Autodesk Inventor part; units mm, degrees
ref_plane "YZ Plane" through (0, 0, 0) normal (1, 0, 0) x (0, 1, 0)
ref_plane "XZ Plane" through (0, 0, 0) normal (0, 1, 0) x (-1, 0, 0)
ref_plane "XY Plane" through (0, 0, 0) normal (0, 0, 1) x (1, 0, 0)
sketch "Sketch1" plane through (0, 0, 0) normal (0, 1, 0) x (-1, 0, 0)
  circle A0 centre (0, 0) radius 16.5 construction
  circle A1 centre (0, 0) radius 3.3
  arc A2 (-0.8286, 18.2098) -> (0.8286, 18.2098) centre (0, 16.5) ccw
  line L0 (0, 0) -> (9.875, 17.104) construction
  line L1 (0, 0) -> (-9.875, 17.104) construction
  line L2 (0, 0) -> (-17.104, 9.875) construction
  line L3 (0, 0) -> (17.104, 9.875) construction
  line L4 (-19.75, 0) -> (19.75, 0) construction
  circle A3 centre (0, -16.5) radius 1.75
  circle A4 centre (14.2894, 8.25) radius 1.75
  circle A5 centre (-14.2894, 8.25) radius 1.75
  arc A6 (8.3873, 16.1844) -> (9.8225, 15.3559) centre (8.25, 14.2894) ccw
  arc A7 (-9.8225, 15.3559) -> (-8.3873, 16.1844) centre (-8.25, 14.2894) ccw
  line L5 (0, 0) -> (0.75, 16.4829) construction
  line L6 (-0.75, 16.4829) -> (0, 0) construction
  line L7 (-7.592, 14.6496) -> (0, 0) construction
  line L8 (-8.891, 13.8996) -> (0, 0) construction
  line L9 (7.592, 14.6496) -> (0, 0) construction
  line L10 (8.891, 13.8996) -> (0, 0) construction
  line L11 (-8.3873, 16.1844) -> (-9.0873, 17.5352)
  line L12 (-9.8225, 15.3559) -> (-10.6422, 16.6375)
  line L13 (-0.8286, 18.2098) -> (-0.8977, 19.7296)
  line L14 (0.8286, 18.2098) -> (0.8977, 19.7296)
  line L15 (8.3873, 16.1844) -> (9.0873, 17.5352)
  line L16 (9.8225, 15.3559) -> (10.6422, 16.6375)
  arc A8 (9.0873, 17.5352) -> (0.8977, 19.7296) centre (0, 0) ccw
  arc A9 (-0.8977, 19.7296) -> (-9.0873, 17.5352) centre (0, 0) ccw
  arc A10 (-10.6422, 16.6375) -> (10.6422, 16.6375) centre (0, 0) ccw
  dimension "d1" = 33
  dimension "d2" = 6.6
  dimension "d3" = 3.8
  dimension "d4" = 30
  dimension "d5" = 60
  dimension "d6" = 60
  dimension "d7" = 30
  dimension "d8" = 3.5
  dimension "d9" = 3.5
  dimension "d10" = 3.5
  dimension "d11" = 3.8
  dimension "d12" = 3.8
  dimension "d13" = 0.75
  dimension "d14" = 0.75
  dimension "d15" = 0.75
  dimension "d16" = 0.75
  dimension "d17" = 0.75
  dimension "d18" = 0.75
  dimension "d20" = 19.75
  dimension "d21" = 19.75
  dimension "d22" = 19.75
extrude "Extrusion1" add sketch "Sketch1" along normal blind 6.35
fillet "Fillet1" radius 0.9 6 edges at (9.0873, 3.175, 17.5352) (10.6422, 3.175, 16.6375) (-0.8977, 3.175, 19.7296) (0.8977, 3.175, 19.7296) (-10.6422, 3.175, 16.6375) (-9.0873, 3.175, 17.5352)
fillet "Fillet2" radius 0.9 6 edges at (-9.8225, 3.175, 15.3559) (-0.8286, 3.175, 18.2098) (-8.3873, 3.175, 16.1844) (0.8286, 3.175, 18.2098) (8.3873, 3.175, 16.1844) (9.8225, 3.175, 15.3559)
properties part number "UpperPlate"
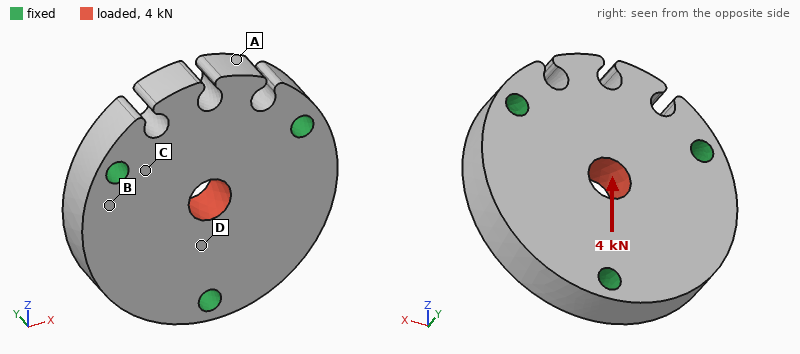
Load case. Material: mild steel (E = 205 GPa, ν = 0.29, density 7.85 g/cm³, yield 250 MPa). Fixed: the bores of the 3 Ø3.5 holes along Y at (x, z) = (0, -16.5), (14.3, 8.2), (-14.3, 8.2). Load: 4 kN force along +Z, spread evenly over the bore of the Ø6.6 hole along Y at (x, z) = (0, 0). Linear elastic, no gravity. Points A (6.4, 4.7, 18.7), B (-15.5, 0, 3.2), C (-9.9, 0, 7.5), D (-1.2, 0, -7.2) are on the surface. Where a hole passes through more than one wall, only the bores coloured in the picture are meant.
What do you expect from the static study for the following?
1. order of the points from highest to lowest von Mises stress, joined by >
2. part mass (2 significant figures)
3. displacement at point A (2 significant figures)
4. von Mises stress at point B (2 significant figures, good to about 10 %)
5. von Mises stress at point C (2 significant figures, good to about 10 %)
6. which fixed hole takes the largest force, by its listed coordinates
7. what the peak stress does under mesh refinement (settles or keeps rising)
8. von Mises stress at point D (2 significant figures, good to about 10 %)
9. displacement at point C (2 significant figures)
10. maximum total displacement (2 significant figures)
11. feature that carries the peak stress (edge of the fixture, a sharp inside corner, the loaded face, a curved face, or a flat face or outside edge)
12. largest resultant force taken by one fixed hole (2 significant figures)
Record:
D > C > B > A
56 g
1.7 µm
13 MPa
21 MPa
(0, -16.5)
keeps rising
32 MPa
0.80 µm
2.8 µm
edge of the fixture
1.6 kN
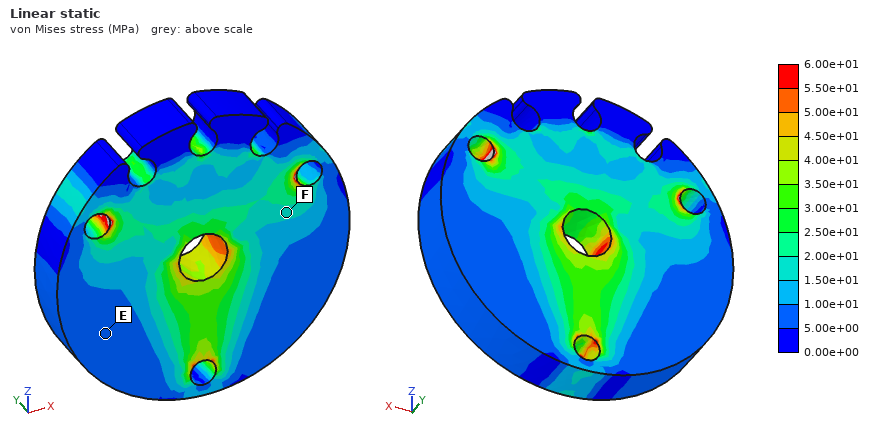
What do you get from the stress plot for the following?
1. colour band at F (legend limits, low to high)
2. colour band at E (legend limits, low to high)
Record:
1.50e+01 to 2.00e+01 MPa
5.00e+00 to 1.00e+01 MPa
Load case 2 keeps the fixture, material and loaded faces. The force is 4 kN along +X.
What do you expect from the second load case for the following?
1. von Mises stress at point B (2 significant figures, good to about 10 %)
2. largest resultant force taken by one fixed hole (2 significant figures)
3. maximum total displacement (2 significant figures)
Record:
14 MPa
1.4 kN
2.3 µm
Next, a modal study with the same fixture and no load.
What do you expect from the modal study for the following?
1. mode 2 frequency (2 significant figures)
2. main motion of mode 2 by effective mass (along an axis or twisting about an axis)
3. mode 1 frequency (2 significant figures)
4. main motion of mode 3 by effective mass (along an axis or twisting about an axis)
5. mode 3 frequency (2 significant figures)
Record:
24 kHz
twisting about Z
22 kHz
along Y
26 kHz
